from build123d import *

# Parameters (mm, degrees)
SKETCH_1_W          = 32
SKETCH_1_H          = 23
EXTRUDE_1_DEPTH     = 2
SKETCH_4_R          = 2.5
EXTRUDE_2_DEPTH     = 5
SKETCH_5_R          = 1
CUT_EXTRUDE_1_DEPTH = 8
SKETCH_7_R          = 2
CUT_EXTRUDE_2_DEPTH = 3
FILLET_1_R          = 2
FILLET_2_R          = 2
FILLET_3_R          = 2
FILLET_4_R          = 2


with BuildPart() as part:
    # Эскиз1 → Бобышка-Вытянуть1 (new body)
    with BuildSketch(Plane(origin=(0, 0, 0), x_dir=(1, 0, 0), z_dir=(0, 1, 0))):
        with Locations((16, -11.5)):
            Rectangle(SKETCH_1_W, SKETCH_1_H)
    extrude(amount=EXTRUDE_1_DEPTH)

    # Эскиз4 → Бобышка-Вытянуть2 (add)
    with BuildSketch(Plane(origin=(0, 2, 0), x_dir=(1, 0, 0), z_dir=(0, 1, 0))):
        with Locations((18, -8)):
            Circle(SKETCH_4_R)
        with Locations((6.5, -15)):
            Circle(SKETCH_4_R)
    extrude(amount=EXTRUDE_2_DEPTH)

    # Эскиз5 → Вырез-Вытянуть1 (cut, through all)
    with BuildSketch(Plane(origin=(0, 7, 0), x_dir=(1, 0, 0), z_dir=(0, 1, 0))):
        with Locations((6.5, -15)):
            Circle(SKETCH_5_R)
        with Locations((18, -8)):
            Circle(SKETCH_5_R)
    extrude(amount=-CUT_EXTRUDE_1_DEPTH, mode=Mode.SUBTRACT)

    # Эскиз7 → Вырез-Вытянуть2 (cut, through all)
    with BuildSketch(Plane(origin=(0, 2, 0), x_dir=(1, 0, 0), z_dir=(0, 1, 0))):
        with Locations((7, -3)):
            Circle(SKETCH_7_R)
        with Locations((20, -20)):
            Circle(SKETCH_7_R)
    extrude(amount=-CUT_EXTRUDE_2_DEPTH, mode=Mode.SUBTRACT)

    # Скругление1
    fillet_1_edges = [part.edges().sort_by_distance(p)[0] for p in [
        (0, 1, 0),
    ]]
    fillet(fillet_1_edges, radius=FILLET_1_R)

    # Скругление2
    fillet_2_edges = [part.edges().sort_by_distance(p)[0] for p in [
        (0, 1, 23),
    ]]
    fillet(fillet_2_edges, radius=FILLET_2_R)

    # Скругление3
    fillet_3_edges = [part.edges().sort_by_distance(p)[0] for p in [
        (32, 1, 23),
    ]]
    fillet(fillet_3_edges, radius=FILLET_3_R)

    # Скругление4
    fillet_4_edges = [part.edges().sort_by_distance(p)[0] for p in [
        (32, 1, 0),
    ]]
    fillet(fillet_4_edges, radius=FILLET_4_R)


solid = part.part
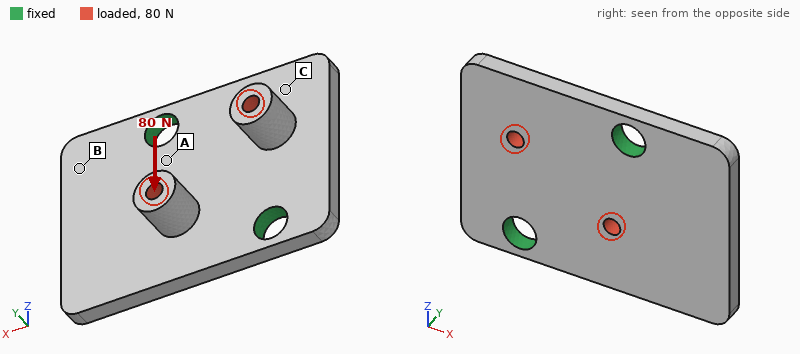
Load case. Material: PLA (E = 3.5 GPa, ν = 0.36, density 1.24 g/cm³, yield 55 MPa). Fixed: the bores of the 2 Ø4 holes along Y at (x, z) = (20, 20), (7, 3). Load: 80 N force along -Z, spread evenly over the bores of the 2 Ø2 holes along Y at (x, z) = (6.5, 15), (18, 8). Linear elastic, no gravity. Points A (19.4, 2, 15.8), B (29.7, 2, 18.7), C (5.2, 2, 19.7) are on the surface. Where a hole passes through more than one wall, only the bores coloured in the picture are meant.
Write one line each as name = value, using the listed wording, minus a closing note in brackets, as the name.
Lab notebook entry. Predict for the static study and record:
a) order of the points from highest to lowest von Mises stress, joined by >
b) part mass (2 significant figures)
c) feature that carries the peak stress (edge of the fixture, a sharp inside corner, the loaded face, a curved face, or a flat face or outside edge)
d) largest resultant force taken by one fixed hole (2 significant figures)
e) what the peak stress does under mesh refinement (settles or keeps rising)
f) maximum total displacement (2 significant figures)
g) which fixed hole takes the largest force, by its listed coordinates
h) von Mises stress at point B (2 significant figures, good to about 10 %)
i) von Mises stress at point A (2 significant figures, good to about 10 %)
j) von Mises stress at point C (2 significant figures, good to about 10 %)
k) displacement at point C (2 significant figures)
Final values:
order of the points from highest to lowest von Mises stress, joined by > = A > C > B
part mass = 1.9 g
feature that carries the peak stress = edge of the fixture
largest resultant force taken by one fixed hole = 45 N
what the peak stress does under mesh refinement = keeps rising
maximum total displacement = 0.15 mm
which fixed hole takes the largest force, by its listed coordinates = (7, 3)
von Mises stress at point B = 1.1 MPa
von Mises stress at point A = 4.5 MPa
von Mises stress at point C = 3.0 MPa
displacement at point C = 0.099 mm
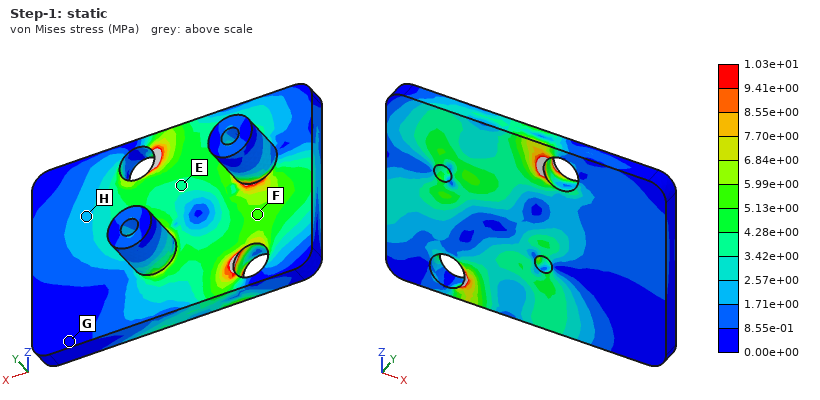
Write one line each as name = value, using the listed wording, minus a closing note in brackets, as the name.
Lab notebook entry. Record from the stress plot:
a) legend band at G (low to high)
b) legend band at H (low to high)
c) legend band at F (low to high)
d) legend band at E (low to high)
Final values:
legend band at G = 0.00e+00 to 8.55e-01 MPa
legend band at H = 1.71e+00 to 2.57e+00 MPa
legend band at F = 5.13e+00 to 5.99e+00 MPa
legend band at E = 3.42e+00 to 4.28e+00 MPa
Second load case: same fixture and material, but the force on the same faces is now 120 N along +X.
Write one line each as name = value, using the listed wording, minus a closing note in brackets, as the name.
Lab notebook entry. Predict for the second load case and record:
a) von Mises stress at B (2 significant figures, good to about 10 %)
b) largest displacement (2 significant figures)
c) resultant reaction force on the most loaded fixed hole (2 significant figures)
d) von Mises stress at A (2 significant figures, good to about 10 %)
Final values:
von Mises stress at B = 2.5 MPa
largest displacement = 0.23 mm
resultant reaction force on the most loaded fixed hole = 61 N
von Mises stress at A = 7.4 MPa
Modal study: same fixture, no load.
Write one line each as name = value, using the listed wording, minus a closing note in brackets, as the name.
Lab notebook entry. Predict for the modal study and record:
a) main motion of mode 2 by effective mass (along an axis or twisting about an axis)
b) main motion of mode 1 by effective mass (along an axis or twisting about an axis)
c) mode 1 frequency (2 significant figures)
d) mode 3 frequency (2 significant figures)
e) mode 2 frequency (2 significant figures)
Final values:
main motion of mode 2 by effective mass = along Y
main motion of mode 1 by effective mass = along Y
mode 1 frequency = 2000 Hz
mode 3 frequency = 5000 Hz
mode 2 frequency = 2800 Hz
